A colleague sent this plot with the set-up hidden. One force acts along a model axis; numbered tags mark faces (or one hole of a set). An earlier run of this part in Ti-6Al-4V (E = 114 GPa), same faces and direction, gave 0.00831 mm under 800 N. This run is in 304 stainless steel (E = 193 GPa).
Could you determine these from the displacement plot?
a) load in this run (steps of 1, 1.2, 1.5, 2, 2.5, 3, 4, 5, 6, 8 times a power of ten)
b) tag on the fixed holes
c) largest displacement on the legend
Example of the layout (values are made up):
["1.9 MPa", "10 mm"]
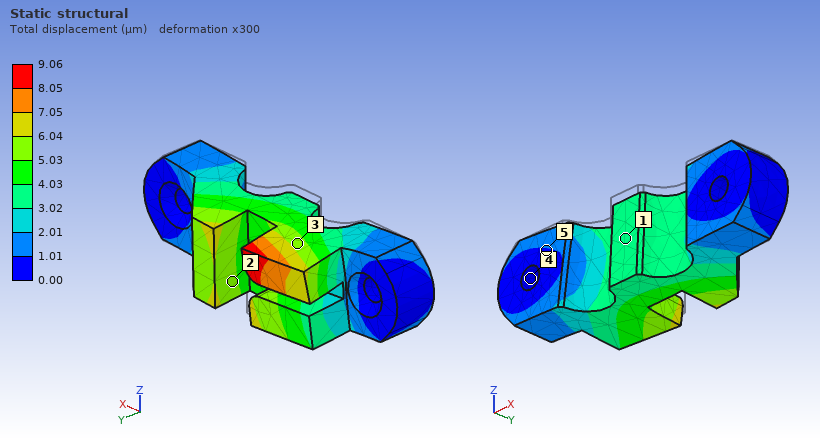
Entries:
["1.5 kN", "4", "9.06 µm"]
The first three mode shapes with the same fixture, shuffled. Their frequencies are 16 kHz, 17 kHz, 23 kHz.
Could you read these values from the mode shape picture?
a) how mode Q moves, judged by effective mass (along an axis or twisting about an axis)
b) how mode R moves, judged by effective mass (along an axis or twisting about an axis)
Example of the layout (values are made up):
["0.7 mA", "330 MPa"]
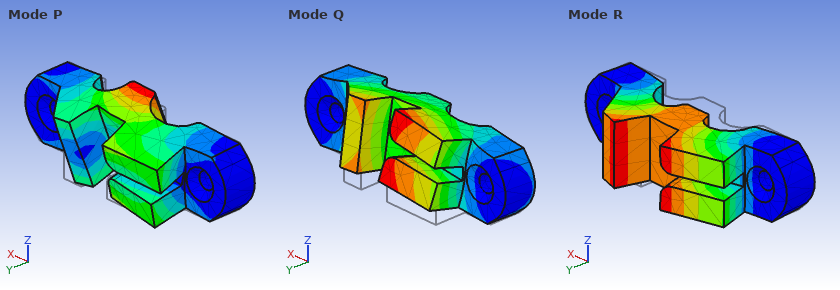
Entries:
["along Z", "along Y"]
